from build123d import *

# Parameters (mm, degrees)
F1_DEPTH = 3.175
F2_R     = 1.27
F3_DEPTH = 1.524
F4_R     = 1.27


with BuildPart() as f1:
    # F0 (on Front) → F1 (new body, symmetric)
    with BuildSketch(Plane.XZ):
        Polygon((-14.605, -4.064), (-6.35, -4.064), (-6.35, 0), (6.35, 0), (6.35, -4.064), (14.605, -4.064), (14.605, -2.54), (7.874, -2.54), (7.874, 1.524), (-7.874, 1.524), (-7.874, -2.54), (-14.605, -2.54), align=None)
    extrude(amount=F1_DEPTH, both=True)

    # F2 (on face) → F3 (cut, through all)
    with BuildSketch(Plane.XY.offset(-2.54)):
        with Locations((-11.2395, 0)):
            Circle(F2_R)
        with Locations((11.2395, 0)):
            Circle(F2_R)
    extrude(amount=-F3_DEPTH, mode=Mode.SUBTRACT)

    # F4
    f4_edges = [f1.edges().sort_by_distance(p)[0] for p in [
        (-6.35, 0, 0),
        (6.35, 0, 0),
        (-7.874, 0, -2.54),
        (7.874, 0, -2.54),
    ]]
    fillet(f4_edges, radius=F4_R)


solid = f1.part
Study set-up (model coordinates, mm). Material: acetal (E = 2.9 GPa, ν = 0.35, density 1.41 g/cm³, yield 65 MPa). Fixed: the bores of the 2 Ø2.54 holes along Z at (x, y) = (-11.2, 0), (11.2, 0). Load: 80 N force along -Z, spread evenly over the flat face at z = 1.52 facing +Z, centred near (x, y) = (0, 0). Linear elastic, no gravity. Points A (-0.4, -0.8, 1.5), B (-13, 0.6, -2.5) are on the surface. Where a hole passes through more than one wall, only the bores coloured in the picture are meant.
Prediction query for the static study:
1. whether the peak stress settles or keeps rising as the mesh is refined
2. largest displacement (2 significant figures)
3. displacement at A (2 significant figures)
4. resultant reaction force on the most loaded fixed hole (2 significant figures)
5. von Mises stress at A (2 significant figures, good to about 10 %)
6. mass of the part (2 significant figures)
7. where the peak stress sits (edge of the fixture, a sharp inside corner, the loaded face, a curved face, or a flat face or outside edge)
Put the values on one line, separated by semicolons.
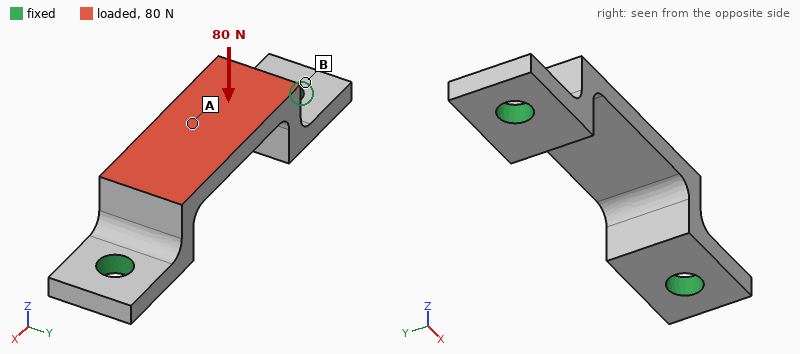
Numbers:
keeps rising; 0.13 mm; 0.12 mm; 57 N; 18 MPa; 0.50 g; edge of the fixture
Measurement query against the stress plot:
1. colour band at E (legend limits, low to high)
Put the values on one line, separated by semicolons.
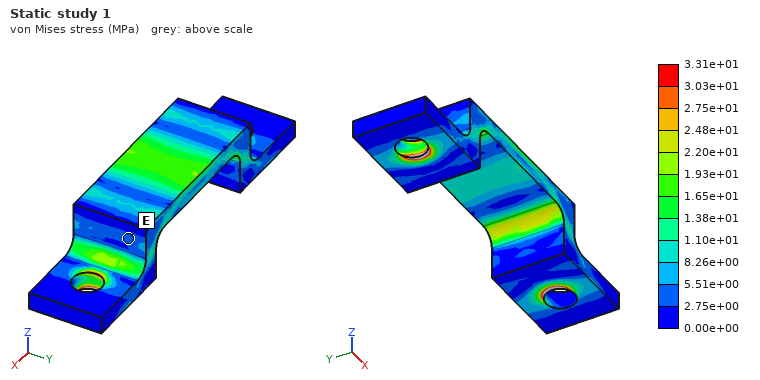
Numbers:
2.75e+00 to 5.51e+00 MPa
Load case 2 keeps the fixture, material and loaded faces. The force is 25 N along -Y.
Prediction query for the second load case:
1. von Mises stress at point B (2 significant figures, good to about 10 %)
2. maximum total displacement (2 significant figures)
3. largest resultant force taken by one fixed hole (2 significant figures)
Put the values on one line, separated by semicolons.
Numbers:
2.8 MPa; 0.11 mm; 13 N
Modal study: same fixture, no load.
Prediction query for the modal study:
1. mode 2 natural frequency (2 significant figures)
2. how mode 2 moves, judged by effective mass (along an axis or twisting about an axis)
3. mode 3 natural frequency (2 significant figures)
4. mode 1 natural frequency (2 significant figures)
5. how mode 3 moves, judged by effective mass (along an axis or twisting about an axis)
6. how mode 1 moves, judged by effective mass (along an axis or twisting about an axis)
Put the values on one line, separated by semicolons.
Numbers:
7600 Hz; along X; 9700 Hz; 5800 Hz; along Z; along Y
